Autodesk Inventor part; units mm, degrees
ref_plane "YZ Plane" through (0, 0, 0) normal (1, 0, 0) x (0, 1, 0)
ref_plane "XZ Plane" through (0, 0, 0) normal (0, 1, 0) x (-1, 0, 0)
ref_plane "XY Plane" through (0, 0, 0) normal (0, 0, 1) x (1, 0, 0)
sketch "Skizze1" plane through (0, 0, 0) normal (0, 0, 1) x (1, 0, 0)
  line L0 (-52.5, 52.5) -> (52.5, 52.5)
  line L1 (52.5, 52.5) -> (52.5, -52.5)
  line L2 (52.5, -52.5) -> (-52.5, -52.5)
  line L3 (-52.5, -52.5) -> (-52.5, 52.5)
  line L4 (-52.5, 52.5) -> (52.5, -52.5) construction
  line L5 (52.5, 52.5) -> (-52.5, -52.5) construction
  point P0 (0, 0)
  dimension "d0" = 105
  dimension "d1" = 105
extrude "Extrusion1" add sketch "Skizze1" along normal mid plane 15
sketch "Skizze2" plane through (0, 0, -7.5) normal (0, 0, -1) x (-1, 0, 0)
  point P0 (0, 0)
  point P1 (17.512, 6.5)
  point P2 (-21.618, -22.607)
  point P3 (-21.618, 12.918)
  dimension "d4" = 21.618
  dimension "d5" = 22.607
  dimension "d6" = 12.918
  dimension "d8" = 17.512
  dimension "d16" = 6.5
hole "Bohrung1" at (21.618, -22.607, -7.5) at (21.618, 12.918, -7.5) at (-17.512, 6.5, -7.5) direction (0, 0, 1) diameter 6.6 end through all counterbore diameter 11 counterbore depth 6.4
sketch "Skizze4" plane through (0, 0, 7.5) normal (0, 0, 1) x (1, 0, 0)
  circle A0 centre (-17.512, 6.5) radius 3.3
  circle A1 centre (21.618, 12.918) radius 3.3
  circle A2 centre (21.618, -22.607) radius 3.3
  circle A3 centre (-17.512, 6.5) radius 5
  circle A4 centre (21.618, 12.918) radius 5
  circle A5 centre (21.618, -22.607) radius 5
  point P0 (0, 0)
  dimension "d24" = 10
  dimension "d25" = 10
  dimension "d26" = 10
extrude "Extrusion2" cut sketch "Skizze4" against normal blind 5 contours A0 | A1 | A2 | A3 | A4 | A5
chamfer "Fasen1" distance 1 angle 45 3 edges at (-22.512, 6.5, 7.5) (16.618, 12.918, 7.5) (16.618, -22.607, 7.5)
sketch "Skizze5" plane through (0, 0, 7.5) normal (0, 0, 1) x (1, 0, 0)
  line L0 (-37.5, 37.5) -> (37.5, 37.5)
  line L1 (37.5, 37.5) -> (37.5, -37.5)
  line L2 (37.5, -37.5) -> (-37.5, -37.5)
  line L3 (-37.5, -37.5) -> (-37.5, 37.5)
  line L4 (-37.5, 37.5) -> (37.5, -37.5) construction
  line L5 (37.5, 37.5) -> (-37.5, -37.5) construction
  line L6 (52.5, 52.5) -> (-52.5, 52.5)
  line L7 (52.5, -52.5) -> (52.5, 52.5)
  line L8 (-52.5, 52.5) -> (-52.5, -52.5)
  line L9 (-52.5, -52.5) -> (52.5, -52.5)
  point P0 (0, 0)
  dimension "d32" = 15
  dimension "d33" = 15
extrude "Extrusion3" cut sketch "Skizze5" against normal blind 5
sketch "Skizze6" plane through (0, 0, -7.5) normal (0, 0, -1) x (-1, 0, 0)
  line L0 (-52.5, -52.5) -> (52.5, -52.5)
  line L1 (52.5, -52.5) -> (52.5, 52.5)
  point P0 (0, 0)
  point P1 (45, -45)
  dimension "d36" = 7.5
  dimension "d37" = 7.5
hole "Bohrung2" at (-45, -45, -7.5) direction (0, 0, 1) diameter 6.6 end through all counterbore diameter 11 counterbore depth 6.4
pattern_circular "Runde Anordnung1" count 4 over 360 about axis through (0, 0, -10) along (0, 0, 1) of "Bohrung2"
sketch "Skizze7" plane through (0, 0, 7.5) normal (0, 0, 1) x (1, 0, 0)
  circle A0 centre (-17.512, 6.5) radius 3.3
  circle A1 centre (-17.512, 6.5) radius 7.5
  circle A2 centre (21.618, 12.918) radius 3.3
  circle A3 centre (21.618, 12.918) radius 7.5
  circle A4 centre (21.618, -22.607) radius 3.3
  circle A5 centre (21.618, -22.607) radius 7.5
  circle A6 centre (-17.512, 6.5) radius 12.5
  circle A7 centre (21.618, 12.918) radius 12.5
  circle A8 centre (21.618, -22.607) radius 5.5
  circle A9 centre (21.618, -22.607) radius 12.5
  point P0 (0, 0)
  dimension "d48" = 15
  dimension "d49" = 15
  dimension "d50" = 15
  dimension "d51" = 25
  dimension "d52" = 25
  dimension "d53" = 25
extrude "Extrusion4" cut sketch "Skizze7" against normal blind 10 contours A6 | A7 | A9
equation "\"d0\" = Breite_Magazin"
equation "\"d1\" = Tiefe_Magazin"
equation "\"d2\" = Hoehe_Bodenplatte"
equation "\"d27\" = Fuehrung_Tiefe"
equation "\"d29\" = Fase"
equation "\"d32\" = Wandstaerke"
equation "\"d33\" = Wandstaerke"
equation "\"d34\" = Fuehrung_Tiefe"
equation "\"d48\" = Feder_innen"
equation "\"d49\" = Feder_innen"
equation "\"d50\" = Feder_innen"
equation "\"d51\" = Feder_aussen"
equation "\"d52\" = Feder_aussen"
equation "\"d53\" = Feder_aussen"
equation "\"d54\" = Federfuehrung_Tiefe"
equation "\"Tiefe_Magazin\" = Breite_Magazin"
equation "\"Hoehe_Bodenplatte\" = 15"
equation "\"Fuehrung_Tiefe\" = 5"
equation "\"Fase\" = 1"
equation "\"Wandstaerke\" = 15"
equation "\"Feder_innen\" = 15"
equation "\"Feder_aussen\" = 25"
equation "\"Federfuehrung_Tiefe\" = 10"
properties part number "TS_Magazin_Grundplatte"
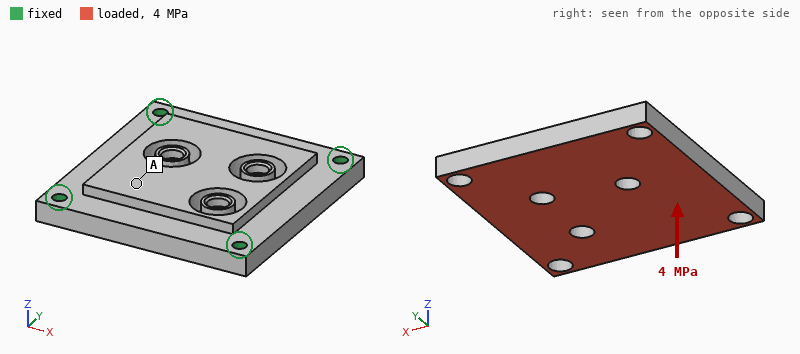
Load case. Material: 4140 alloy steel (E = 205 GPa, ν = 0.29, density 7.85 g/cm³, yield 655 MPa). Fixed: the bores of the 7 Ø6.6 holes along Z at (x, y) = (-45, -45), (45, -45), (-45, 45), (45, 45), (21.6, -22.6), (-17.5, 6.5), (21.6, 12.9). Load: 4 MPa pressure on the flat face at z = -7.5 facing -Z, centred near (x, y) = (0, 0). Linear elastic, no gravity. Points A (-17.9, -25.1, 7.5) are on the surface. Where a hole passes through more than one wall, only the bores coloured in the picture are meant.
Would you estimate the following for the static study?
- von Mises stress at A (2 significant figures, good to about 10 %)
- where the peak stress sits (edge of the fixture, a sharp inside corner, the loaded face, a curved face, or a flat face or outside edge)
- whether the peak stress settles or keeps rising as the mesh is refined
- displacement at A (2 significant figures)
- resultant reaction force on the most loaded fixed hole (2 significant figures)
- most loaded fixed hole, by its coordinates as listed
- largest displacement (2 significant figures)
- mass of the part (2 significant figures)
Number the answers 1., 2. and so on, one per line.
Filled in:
1. 33 MPa
2. edge of the fixture
3. keeps rising
4. 20 µm
5. 9.7 kN
6. (-17.5, 6.5)
7. 31 µm
8. 960 g
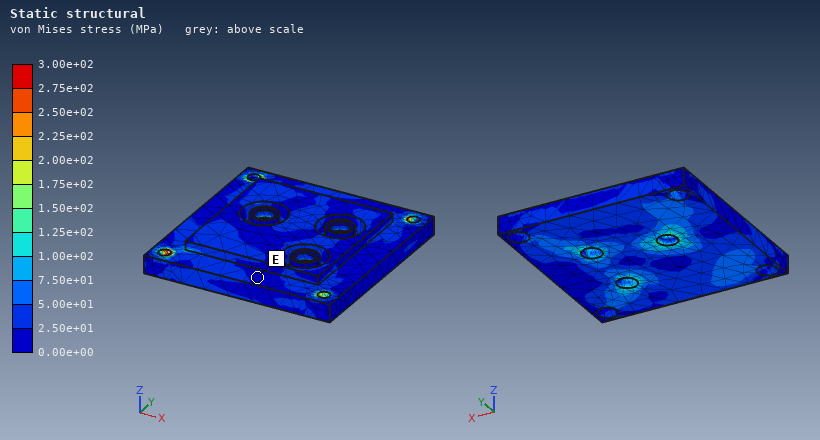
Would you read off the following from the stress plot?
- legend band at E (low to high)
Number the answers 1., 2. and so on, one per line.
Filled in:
1. 0.00e+00 to 2.50e+01 MPa
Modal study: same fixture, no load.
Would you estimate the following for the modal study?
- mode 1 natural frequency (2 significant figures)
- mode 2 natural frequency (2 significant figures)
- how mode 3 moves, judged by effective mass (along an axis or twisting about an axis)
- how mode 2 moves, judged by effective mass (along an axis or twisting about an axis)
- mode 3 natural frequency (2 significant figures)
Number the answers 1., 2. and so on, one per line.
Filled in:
1. 6700 Hz
2. 7000 Hz
3. along Z
4. along Z
5. 7900 Hz
